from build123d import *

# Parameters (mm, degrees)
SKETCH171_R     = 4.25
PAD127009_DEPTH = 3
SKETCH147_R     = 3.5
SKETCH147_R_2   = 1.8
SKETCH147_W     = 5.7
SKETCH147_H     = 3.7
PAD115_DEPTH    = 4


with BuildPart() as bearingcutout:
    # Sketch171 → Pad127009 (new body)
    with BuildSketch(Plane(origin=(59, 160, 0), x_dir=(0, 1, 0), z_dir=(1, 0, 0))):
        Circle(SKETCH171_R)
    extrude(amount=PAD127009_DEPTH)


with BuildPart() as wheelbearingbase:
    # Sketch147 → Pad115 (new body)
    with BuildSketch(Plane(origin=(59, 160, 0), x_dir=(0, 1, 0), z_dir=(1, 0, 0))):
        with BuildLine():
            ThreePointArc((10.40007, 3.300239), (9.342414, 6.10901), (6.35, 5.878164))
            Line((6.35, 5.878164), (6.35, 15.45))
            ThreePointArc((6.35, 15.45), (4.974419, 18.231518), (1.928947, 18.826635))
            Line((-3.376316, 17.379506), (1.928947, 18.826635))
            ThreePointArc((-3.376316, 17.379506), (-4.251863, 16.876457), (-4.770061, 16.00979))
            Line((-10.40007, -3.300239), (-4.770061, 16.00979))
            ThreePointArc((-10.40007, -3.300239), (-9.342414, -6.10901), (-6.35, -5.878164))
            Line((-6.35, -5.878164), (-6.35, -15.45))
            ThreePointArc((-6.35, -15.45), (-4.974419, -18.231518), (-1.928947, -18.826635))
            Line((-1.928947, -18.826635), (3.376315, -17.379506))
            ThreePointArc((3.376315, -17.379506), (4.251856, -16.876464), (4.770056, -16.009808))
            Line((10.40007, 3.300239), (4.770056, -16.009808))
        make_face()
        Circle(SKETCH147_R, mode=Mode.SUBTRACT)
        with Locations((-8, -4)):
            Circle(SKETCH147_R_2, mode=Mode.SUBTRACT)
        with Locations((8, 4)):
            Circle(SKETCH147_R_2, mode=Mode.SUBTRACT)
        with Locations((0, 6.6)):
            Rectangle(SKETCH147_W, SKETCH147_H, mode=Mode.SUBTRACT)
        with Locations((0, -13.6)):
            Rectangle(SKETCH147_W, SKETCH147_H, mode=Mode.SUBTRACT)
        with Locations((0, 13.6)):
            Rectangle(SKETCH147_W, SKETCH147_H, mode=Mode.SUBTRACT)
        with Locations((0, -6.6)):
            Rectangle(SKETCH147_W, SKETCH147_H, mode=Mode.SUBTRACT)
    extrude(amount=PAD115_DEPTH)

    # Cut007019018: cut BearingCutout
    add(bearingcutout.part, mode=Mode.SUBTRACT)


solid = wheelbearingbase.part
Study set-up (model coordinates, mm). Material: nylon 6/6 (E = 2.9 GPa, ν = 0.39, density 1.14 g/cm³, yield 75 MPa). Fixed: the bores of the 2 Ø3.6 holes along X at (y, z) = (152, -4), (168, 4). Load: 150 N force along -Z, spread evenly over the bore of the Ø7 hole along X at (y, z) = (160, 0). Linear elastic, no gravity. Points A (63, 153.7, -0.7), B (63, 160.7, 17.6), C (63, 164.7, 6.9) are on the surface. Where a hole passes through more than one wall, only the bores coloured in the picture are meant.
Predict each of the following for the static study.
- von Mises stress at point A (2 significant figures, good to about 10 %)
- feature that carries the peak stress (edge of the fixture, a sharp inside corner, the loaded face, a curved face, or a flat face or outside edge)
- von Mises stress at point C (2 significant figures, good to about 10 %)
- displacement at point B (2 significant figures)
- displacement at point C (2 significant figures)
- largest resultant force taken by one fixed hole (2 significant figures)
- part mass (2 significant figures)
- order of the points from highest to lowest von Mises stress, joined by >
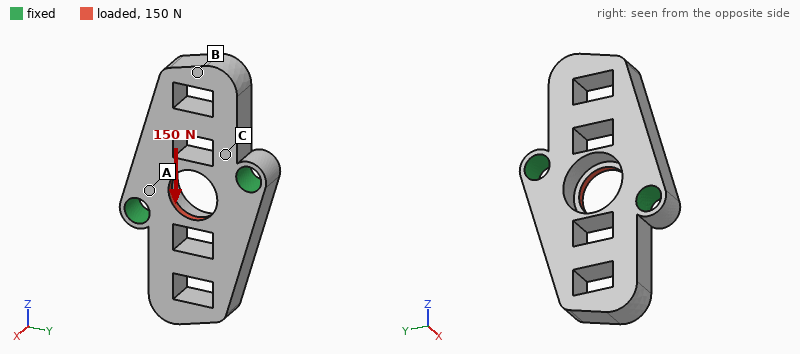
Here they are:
5.8 MPa
the loaded face
4.2 MPa
37 µm
9.4 µm
75 N
1.7 g
A > C > B
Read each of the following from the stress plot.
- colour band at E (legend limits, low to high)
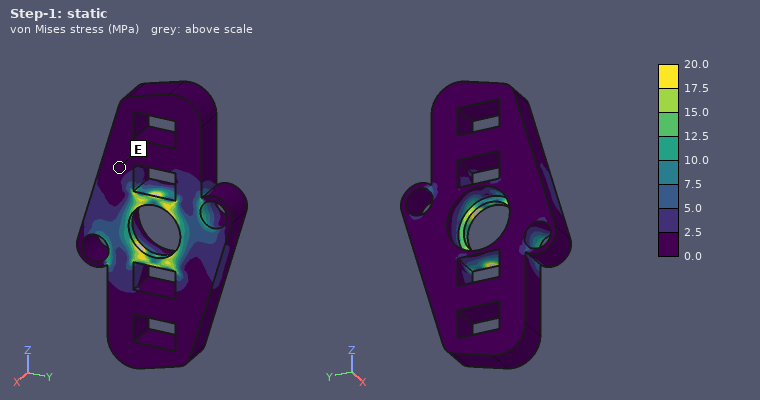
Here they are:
0.0 to 2.5 MPa
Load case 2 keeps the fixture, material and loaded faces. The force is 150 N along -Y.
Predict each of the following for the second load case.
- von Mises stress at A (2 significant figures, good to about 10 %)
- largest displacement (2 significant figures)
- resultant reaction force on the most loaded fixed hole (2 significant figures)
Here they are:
6.0 MPa
21 µm
75 N
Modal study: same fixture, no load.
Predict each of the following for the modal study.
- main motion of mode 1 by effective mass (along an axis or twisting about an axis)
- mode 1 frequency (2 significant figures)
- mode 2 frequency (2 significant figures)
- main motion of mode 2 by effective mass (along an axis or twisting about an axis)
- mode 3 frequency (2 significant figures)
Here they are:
twisting about Y
3300 Hz
3500 Hz
along X
7600 Hz
